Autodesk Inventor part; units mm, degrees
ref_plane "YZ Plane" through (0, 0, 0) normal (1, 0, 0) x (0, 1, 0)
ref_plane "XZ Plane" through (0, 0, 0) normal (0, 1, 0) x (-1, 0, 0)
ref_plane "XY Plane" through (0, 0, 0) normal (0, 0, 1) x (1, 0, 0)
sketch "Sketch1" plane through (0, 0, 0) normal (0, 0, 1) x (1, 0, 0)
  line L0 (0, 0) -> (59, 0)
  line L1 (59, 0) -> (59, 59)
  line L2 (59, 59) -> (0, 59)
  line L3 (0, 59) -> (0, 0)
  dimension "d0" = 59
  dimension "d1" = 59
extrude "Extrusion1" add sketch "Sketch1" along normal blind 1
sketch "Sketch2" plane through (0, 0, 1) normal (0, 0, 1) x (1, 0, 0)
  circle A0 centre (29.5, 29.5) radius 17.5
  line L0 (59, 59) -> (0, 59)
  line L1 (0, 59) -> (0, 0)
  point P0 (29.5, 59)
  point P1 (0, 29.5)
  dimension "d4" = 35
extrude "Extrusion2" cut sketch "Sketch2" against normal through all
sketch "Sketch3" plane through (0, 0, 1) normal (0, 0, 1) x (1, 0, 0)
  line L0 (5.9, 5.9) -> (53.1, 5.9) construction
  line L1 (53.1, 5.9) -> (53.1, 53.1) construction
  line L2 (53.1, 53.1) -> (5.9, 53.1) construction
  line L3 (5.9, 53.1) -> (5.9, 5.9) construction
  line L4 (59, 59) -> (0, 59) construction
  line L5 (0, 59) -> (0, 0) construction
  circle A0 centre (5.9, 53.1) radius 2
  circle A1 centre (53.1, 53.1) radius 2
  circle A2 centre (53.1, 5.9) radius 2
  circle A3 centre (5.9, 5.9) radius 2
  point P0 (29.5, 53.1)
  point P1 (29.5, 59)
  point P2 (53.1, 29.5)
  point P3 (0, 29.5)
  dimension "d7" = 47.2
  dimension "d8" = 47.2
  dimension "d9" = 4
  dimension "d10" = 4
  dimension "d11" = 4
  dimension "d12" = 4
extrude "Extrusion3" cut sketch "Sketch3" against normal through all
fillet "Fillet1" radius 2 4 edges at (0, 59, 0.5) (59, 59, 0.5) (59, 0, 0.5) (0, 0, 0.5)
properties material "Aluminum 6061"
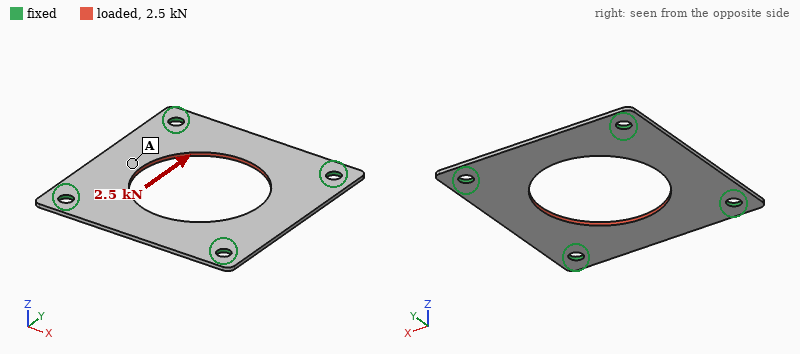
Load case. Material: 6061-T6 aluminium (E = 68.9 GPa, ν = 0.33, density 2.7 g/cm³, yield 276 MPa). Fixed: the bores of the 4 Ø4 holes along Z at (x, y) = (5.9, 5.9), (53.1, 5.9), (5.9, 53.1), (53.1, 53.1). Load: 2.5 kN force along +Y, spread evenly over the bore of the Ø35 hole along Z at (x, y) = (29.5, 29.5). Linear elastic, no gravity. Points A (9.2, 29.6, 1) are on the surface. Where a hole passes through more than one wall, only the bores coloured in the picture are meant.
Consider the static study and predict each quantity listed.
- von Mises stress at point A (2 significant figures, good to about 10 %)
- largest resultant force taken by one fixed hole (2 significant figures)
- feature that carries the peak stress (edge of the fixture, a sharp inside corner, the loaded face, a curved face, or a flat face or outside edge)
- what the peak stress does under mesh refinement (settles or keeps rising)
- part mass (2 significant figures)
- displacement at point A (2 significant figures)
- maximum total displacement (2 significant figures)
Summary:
47 MPa
650 N
edge of the fixture
keeps rising
6.7 g
10 µm
31 µm
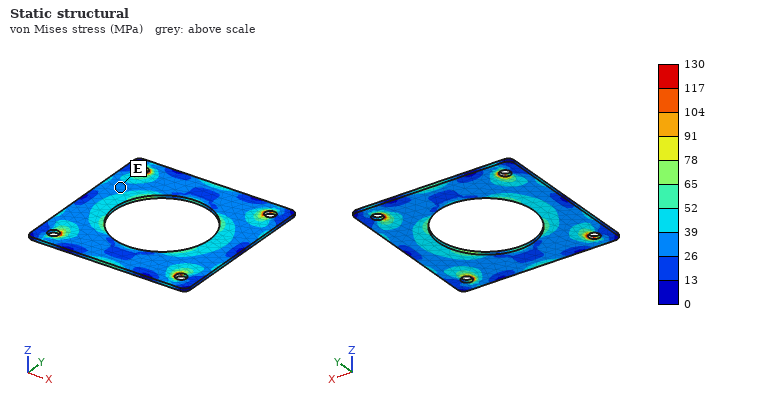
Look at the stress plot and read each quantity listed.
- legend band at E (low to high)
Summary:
26 to 39 MPa
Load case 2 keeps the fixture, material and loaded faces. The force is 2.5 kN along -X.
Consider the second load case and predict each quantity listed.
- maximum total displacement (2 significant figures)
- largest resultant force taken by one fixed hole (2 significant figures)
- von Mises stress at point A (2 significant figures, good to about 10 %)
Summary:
31 µm
650 N
21 MPa
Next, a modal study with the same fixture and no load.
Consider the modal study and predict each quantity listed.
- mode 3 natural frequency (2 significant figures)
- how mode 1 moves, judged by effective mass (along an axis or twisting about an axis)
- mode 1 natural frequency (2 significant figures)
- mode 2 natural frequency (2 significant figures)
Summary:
2800 Hz
along Z
2600 Hz
2800 Hz
